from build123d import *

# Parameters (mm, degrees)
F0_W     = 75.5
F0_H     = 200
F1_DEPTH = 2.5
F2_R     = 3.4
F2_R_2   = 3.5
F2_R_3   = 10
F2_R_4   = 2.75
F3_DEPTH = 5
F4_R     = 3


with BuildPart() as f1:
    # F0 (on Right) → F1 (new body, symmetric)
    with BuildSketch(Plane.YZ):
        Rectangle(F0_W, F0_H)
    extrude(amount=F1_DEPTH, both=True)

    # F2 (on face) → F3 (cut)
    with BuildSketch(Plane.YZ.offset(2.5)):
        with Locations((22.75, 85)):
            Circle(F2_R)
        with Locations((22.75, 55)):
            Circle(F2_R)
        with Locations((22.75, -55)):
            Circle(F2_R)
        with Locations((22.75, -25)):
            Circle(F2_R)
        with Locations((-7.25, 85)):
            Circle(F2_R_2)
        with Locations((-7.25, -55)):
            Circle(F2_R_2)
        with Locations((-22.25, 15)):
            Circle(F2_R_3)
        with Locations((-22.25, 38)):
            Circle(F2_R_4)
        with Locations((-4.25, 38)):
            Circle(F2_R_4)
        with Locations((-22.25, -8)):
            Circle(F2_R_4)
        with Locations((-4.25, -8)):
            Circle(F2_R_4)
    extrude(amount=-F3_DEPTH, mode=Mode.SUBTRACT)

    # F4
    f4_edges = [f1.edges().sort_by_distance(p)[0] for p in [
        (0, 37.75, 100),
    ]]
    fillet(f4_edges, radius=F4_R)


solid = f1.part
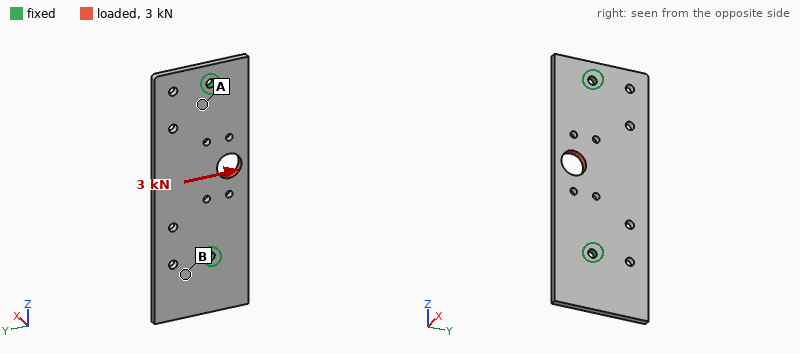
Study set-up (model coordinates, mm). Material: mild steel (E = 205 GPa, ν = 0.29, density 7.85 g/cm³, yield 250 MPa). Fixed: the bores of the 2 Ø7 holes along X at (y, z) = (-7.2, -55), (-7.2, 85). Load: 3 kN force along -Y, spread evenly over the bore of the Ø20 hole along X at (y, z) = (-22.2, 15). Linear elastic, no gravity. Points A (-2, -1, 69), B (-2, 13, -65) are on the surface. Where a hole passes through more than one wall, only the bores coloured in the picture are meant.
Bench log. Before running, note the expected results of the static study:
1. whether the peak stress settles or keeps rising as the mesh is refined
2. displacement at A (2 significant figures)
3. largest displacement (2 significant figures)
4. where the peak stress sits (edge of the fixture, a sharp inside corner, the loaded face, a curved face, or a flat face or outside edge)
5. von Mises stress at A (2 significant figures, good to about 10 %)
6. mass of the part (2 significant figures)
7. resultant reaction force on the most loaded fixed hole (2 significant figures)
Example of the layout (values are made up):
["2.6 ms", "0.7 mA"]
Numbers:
["keeps rising", "2.7 µm", "11 µm", "edge of the fixture", "12 MPa", "570 g", "1.6 kN"]
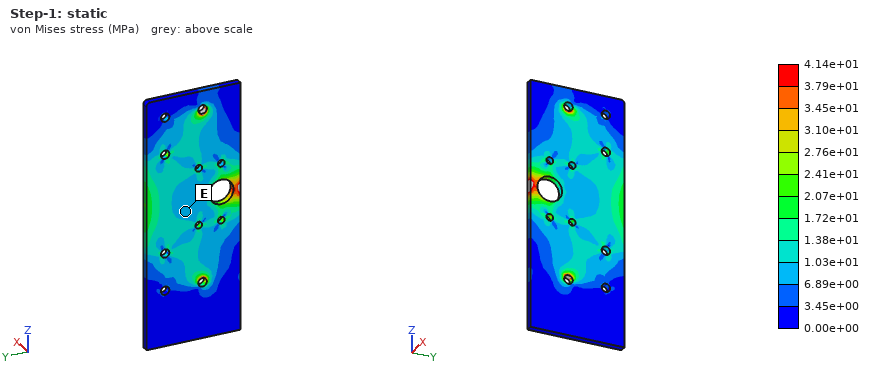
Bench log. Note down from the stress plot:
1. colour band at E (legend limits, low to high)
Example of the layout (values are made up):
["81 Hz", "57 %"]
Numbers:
["6.89e+00 to 1.03e+01 MPa"]
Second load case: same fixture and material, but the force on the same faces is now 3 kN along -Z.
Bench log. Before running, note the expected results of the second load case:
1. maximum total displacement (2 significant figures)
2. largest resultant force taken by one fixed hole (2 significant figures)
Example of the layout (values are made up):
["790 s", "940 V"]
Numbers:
["3.6 µm", "1.6 kN"]
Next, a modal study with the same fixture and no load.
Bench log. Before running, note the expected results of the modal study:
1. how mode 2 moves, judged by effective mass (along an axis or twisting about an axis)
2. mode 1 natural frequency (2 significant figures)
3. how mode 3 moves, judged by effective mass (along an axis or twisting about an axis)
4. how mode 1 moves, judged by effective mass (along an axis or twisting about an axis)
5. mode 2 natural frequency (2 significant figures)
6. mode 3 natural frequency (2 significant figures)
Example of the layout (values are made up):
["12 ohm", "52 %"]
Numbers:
["twisting about Z", "1000 Hz", "along X", "along X", "1400 Hz", "1600 Hz"]
